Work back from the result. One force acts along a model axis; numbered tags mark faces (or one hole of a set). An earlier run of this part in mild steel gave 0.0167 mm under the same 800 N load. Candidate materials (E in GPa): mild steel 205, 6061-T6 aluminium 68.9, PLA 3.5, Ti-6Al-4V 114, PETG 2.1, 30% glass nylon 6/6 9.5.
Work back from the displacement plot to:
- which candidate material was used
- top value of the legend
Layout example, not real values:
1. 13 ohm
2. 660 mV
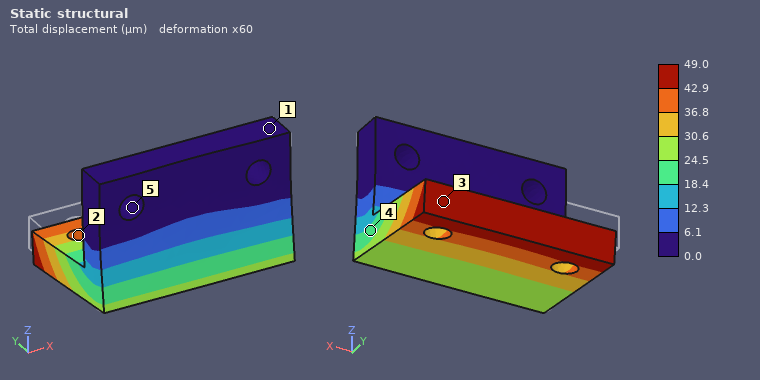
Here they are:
1. 6061-T6 aluminium
2. 49.0 µm
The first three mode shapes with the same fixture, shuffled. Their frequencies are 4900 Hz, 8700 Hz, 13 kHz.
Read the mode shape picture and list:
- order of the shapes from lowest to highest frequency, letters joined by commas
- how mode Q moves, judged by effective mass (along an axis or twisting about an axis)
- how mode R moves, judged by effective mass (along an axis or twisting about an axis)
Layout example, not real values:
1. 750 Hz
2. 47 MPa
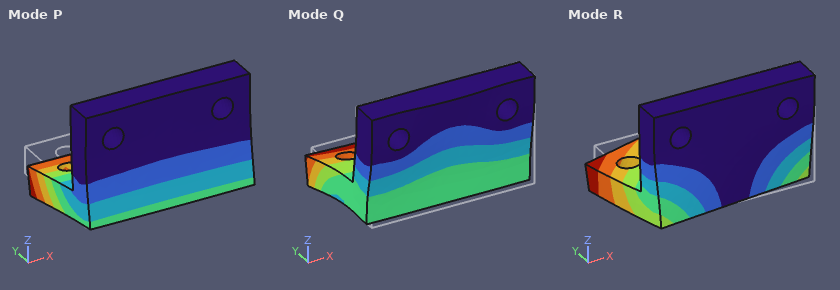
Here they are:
1. P, R, Q
2. along Y
3. along X
